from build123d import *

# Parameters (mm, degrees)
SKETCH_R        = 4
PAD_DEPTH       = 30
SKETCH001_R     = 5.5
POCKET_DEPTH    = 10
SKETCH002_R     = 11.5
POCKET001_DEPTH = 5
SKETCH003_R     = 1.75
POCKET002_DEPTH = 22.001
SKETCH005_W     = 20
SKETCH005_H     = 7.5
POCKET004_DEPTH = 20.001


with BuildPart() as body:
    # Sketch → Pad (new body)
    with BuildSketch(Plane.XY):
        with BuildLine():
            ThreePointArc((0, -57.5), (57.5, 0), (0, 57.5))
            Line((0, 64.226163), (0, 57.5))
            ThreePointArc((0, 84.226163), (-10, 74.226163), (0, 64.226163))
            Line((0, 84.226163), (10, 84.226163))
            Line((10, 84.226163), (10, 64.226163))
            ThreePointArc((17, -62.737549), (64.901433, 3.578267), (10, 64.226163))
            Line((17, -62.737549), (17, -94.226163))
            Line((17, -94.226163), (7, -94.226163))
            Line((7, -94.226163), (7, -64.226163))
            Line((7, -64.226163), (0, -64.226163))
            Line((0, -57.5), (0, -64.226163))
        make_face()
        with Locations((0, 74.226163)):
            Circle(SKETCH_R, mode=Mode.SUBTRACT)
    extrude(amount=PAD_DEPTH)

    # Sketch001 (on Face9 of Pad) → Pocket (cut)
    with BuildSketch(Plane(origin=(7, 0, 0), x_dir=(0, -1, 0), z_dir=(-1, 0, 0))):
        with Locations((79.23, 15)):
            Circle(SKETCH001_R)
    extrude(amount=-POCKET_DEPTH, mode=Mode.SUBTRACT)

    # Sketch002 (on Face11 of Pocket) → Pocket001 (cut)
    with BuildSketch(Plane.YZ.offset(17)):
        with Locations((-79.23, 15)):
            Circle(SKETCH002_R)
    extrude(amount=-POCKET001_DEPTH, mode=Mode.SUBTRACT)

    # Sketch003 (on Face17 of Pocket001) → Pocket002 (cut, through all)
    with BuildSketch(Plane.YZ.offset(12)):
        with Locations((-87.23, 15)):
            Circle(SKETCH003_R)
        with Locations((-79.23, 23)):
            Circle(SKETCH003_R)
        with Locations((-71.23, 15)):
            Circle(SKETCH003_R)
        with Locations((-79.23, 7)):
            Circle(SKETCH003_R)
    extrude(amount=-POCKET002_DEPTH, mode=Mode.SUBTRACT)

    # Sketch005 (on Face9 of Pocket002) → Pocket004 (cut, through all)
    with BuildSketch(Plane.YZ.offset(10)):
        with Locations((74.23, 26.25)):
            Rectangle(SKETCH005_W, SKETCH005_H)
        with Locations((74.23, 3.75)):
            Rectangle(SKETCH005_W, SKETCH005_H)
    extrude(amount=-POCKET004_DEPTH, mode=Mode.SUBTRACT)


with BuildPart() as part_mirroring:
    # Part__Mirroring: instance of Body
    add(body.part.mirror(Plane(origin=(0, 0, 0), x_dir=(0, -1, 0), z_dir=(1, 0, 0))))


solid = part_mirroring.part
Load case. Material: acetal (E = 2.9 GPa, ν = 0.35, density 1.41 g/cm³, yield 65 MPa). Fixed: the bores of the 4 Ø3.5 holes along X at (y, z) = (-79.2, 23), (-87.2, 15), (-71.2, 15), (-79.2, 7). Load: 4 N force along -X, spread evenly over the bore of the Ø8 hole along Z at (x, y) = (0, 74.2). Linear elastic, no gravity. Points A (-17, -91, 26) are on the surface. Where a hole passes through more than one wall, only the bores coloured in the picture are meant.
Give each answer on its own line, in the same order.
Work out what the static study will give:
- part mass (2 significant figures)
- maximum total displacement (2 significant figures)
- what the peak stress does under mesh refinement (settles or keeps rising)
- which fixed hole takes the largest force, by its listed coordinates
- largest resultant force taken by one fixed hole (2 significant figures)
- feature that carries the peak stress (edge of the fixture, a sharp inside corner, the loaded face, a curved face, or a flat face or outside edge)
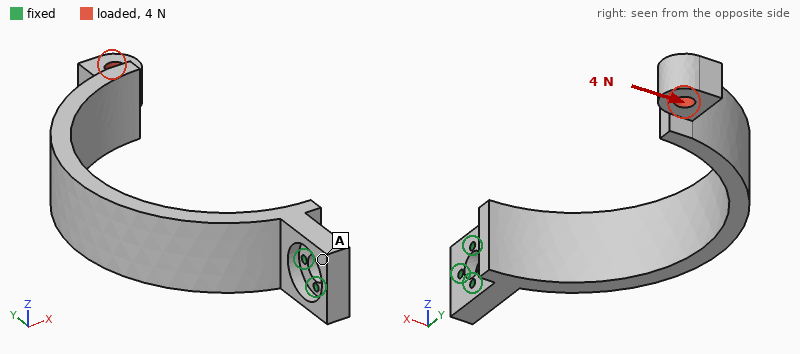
76 g
2.1 mm
keeps rising
(-71.2, 15)
38 N
edge of the fixture
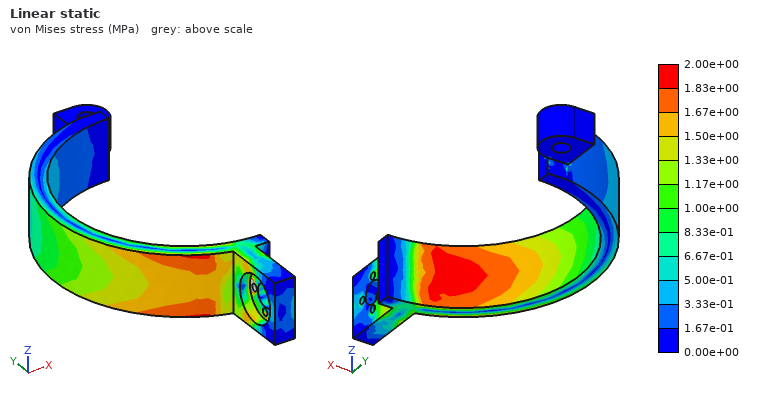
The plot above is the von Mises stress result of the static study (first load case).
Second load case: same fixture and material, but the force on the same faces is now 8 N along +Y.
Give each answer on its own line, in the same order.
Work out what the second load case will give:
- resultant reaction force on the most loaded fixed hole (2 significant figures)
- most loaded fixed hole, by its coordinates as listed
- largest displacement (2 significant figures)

7.0 N
(-71.2, 15)
1.9 mm
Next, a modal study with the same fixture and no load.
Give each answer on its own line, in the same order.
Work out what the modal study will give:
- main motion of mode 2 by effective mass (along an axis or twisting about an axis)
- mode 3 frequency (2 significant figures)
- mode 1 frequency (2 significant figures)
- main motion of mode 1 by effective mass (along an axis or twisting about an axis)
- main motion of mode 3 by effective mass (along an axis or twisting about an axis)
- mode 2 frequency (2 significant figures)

along Z
150 Hz
49 Hz
along X
along Y
76 Hz
